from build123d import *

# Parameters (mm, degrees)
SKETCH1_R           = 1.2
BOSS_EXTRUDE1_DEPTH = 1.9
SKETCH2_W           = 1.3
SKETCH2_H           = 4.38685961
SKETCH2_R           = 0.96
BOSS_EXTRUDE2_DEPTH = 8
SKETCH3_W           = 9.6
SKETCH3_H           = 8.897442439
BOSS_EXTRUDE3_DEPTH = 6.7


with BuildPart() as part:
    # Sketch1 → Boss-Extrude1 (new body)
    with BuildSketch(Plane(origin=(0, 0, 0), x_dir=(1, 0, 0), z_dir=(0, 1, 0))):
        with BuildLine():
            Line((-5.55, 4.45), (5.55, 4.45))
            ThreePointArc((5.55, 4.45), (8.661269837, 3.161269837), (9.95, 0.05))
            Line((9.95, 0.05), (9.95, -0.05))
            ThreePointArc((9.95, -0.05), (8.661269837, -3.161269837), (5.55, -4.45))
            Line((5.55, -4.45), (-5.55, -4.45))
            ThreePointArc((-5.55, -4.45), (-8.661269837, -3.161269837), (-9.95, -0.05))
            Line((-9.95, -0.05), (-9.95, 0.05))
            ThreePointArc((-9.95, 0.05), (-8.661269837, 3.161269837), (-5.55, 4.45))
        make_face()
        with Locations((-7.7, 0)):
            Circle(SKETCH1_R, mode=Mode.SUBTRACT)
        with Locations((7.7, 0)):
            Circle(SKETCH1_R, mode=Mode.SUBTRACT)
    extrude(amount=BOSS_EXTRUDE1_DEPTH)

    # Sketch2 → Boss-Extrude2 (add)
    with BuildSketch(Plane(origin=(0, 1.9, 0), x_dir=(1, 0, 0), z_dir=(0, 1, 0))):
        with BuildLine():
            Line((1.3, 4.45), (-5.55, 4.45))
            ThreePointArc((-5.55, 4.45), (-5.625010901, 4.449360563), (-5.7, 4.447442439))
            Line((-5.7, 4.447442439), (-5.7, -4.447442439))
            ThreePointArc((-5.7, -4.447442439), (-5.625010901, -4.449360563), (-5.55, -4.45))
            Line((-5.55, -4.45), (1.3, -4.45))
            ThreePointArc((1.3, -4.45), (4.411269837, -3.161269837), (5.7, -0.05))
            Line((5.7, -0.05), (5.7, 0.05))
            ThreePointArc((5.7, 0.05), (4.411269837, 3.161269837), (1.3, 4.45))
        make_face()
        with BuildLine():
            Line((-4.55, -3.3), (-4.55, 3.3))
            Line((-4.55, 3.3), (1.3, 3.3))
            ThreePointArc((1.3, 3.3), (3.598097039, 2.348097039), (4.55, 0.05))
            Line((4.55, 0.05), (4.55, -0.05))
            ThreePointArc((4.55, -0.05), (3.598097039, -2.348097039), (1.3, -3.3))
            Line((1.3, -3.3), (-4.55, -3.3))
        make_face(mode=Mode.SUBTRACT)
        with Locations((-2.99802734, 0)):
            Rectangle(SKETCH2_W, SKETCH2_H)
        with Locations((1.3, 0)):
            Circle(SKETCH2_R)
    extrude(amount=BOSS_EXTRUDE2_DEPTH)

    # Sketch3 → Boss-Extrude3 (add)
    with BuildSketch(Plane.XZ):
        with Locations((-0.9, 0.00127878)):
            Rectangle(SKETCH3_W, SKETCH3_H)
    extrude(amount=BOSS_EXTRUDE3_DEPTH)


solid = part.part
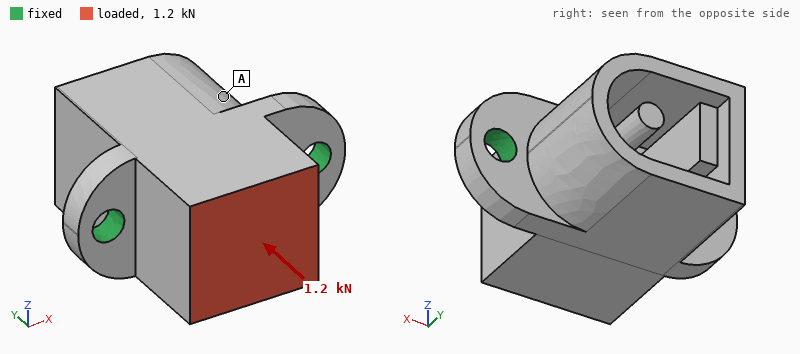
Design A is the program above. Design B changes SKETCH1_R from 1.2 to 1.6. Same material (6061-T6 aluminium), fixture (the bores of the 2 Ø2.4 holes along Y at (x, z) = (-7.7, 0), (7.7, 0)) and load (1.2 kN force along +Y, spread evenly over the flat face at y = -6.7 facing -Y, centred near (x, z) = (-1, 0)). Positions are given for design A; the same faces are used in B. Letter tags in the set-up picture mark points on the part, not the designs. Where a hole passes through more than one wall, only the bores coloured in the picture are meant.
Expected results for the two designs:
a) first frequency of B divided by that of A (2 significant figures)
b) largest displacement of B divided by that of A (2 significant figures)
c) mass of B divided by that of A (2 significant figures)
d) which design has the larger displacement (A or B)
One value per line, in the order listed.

1.2
0.79
0.99
A
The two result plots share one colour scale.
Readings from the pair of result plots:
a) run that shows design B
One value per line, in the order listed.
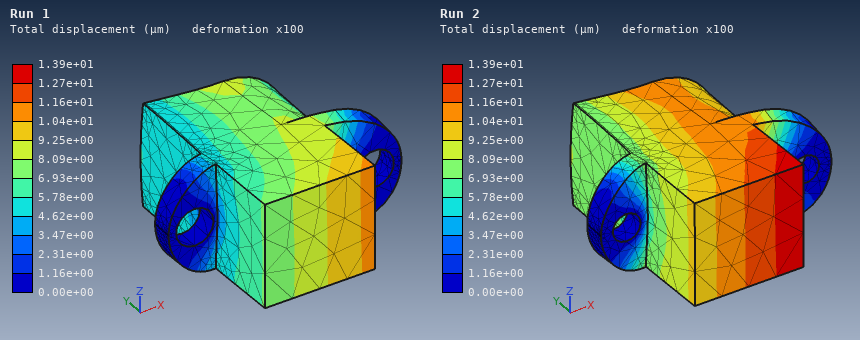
Run 1
